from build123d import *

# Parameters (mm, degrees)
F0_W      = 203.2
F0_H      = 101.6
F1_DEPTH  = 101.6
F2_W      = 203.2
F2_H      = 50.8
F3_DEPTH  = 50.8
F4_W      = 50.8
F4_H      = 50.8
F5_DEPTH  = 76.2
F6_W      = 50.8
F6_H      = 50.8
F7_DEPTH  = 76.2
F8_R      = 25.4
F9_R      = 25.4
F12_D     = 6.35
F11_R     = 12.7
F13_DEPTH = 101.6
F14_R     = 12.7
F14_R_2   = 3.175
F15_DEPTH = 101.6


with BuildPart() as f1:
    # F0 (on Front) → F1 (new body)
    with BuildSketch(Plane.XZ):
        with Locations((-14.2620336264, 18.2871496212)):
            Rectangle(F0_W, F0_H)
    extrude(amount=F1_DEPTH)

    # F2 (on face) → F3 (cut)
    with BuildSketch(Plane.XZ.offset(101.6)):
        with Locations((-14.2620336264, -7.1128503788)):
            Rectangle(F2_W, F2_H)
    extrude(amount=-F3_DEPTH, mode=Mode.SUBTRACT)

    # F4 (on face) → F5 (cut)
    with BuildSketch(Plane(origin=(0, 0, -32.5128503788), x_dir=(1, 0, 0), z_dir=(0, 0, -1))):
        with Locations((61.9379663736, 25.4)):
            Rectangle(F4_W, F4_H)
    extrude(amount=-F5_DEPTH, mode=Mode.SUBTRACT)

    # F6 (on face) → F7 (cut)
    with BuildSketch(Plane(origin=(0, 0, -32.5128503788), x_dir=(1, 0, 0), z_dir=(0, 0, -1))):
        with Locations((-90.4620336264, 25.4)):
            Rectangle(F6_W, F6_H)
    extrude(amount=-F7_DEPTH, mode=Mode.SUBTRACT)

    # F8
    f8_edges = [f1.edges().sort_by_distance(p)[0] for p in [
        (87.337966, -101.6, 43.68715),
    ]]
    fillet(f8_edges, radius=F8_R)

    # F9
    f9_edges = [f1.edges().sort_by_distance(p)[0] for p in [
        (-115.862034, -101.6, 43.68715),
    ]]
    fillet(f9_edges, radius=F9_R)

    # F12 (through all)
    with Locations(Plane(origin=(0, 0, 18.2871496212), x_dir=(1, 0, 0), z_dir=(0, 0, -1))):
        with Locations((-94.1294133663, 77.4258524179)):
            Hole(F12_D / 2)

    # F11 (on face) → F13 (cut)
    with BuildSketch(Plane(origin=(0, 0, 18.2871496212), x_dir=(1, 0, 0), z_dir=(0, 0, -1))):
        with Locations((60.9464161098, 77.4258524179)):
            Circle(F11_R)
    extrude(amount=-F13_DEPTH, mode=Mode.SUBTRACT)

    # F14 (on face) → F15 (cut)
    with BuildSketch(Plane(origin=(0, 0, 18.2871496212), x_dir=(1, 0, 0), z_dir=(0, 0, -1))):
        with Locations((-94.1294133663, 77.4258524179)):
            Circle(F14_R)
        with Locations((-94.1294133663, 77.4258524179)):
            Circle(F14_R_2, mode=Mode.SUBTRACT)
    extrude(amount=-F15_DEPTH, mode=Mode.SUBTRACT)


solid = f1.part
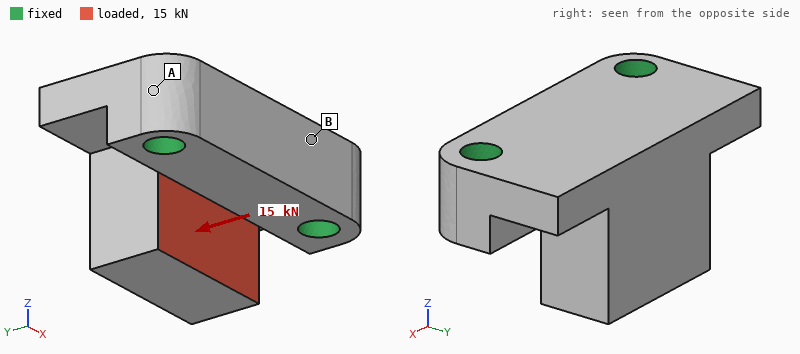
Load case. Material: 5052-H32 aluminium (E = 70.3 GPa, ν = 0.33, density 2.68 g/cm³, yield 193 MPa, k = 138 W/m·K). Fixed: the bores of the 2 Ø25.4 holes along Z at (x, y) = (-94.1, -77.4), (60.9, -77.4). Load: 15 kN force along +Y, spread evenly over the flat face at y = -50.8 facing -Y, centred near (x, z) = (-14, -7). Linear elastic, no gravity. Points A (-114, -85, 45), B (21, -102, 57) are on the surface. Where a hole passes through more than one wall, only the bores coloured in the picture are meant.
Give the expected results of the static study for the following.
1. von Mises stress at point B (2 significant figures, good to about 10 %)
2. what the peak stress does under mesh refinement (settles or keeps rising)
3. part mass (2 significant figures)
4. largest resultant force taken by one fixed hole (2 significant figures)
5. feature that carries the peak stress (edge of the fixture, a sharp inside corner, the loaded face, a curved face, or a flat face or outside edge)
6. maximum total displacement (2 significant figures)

8.4 MPa
keeps rising
3.0 kg
8.5 kN
a sharp inside corner
72 µm
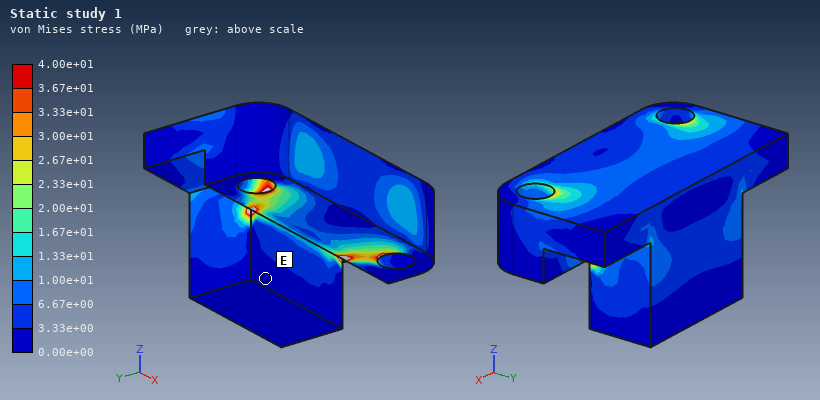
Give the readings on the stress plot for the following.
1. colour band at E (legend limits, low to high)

0.00e+00 to 3.33e+00 MPa
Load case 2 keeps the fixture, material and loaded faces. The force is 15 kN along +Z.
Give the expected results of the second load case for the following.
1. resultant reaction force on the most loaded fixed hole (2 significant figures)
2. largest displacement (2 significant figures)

7.8 kN
17 µm
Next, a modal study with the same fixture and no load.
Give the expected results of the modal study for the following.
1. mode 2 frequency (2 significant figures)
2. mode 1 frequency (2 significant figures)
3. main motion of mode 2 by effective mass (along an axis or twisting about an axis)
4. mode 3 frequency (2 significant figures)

4700 Hz
2400 Hz
along X
5400 Hz
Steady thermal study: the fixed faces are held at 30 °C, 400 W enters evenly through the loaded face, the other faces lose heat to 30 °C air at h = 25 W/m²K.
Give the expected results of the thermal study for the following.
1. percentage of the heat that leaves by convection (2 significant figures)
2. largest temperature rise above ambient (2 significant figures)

8.3 %
54 K
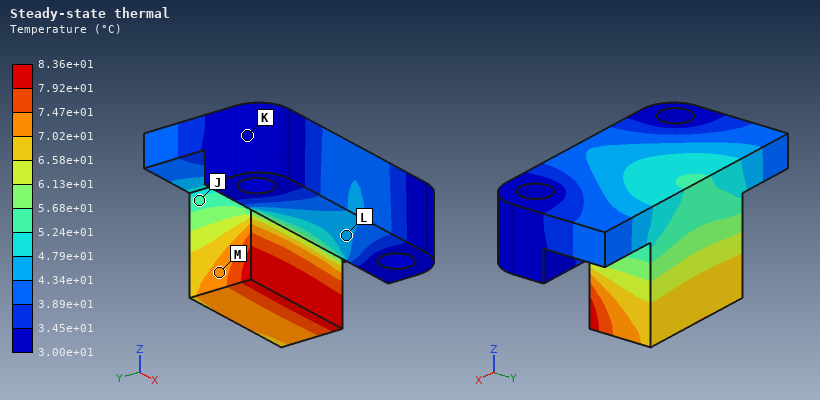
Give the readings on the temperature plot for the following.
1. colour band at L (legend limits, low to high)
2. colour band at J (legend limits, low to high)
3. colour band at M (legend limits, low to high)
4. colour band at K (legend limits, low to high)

4.34e+01 to 4.79e+01 °C
5.24e+01 to 5.68e+01 °C
7.02e+01 to 7.47e+01 °C
3.00e+01 to 3.45e+01 °C
